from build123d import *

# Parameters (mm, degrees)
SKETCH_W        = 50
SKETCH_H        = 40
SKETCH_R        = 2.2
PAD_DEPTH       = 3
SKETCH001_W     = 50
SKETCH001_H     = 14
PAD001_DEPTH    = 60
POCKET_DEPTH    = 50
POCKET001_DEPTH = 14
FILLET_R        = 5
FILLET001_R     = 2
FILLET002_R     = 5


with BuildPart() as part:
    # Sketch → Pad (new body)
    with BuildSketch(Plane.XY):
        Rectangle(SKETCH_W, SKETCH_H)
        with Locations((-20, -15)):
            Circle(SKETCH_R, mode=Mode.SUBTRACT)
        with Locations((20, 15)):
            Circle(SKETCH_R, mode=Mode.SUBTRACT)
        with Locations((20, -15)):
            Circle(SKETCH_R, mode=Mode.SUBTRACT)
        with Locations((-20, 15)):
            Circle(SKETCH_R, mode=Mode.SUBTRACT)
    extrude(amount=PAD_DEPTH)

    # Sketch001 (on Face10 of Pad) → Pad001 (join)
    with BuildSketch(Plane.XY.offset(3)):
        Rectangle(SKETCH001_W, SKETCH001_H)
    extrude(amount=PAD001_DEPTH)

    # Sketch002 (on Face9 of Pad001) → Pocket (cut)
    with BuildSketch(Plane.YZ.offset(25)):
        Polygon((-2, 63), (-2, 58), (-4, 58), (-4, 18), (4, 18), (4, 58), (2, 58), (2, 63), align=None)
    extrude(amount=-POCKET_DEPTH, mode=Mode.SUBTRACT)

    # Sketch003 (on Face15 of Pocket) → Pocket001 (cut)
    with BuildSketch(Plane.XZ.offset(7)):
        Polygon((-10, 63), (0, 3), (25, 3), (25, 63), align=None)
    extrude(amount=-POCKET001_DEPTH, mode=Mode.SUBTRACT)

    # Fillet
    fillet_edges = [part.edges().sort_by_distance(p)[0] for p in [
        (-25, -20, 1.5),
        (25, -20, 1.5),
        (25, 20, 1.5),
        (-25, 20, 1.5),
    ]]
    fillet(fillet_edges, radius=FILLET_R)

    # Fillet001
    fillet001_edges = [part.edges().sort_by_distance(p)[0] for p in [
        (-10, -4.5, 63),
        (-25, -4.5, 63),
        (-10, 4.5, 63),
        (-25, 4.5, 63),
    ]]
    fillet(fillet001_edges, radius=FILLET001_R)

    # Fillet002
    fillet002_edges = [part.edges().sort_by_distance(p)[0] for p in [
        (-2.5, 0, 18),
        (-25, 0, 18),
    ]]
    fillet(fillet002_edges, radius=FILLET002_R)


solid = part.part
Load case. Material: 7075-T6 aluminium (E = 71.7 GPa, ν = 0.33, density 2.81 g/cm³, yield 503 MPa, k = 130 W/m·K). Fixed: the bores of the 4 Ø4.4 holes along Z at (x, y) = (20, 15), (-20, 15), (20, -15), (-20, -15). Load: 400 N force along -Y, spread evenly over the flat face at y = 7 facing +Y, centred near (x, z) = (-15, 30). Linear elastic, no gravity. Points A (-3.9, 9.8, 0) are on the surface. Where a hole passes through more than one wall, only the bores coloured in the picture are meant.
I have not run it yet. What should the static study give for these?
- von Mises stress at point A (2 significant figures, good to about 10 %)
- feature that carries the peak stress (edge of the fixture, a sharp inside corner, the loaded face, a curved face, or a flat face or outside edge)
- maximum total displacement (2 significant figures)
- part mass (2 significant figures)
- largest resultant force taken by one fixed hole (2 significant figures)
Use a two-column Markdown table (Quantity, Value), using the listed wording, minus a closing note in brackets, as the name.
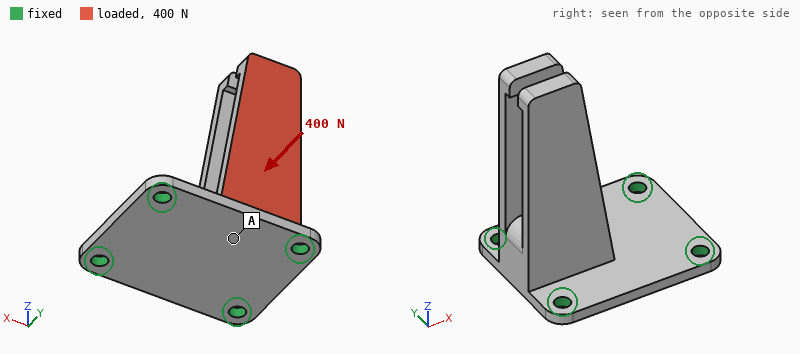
| Quantity | Value |
|---|---|
| von Mises stress at point A | 19 MPa |
| feature that carries the peak stress | the loaded face |
| maximum total displacement | 1.1 mm |
| part mass | 45 g |
| largest resultant force taken by one fixed hole | 500 N |
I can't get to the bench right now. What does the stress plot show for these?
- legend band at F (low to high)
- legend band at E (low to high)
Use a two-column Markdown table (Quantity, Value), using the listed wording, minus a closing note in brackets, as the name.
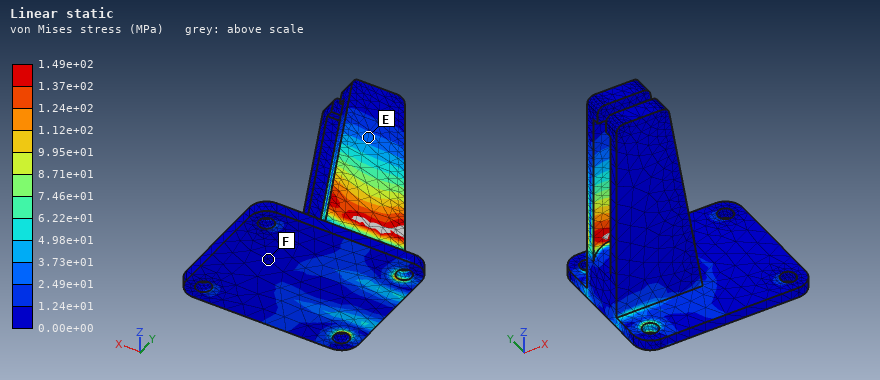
| Quantity | Value |
|---|---|
| legend band at F | 0.00e+00 to 1.24e+01 MPa |
| legend band at E | 2.49e+01 to 3.73e+01 MPa |
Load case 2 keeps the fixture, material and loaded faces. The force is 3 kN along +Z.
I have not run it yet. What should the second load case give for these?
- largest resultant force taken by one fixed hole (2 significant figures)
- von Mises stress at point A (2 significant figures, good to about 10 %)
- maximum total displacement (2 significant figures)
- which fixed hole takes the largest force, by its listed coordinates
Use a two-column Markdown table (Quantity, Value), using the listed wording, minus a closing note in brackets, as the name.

| Quantity | Value |
|---|---|
| largest resultant force taken by one fixed hole | 2.2 kN |
| von Mises stress at point A | 82 MPa |
| maximum total displacement | 0.87 mm |
| which fixed hole takes the largest force, by its listed coordinates | (-20, 15) |
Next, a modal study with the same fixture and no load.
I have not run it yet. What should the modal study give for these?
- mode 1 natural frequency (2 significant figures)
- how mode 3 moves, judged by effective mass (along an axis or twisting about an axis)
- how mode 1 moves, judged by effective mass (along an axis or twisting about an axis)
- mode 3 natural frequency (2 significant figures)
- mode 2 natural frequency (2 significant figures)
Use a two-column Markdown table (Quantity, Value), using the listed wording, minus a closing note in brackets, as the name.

| Quantity | Value |
|---|---|
| mode 1 natural frequency | 1100 Hz |
| how mode 3 moves, judged by effective mass | along X |
| how mode 1 moves, judged by effective mass | along Y |
| mode 3 natural frequency | 2000 Hz |
| mode 2 natural frequency | 1200 Hz |
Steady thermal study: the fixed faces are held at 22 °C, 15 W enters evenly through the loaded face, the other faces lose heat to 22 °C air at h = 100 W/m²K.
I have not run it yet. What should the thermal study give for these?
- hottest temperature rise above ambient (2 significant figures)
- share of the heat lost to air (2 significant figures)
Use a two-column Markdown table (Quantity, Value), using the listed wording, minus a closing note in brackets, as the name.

| Quantity | Value |
|---|---|
| hottest temperature rise above ambient | 30 K |
| share of the heat lost to air | 37 % |
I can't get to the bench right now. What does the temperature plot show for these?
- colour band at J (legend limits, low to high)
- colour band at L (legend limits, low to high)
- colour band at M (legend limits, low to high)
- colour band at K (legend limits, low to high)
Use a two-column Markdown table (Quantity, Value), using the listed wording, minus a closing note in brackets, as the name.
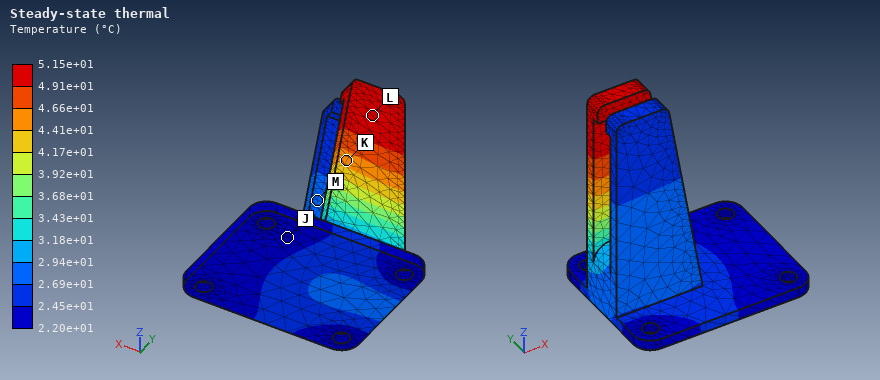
| Quantity | Value |
|---|---|
| colour band at J | 2.20e+01 to 2.45e+01 °C |
| colour band at L | 4.91e+01 to 5.15e+01 °C |
| colour band at M | 2.69e+01 to 2.94e+01 °C |
| colour band at K | 4.41e+01 to 4.66e+01 °C |
